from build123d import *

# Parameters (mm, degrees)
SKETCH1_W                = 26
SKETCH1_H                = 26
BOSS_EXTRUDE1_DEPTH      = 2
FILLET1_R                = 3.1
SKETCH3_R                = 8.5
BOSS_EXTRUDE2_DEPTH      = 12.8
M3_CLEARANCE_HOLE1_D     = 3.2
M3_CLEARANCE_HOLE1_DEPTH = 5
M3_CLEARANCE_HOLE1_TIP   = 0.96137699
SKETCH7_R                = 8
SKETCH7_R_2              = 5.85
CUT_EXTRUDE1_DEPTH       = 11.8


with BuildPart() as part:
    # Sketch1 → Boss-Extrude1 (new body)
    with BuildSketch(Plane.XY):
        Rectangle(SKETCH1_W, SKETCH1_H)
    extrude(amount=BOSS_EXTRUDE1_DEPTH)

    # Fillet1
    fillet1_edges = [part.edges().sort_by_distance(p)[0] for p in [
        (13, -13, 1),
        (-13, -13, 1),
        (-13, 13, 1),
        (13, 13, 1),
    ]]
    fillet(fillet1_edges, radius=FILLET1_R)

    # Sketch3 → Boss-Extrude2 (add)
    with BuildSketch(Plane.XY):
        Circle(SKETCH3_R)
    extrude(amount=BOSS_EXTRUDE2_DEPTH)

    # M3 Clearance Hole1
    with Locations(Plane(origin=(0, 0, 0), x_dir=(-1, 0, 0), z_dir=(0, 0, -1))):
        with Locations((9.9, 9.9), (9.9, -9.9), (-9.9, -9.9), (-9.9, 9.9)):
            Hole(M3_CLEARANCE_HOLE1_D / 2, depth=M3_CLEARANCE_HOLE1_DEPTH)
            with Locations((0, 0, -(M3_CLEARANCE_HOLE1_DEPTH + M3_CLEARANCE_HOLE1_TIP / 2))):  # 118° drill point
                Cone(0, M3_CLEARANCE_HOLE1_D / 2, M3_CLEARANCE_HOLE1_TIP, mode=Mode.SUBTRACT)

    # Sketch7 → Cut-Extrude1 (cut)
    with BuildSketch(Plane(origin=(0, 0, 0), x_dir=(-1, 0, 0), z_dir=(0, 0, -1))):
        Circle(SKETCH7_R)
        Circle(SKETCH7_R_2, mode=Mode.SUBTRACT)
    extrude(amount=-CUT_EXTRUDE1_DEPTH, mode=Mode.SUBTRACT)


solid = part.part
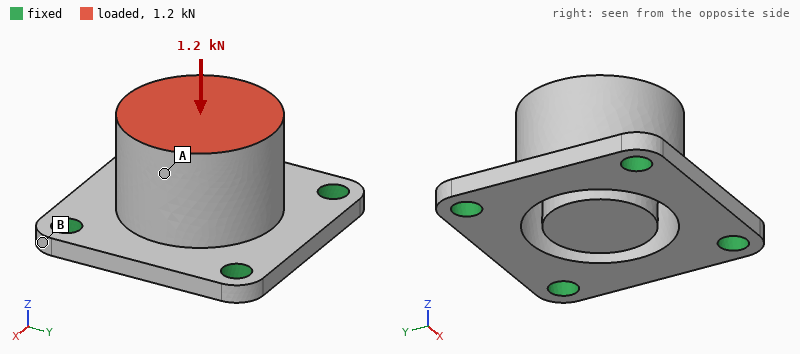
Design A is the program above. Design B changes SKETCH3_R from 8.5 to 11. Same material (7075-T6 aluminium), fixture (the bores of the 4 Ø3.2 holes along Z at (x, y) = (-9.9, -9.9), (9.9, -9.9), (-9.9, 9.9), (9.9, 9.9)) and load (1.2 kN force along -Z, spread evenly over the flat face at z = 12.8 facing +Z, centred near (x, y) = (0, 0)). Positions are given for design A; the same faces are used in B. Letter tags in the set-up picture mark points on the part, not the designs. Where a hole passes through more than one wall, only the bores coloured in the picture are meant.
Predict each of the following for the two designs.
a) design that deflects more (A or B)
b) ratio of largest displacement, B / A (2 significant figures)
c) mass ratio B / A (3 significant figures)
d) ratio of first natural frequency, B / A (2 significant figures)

A
0.24
1.63
1.4
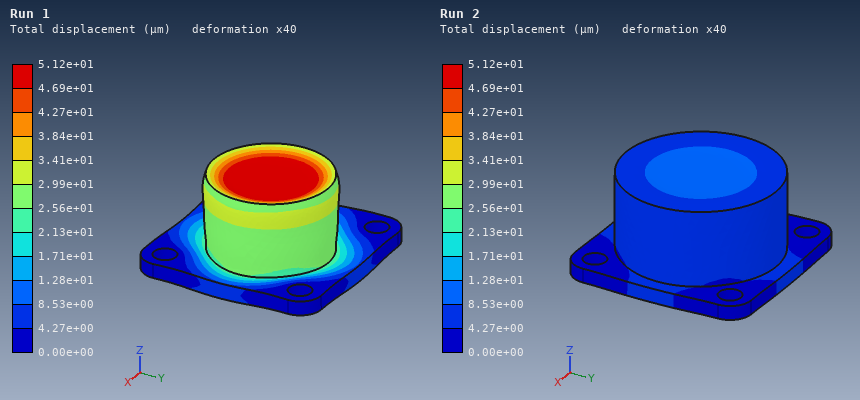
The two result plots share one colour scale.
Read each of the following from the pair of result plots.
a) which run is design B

Run 2
